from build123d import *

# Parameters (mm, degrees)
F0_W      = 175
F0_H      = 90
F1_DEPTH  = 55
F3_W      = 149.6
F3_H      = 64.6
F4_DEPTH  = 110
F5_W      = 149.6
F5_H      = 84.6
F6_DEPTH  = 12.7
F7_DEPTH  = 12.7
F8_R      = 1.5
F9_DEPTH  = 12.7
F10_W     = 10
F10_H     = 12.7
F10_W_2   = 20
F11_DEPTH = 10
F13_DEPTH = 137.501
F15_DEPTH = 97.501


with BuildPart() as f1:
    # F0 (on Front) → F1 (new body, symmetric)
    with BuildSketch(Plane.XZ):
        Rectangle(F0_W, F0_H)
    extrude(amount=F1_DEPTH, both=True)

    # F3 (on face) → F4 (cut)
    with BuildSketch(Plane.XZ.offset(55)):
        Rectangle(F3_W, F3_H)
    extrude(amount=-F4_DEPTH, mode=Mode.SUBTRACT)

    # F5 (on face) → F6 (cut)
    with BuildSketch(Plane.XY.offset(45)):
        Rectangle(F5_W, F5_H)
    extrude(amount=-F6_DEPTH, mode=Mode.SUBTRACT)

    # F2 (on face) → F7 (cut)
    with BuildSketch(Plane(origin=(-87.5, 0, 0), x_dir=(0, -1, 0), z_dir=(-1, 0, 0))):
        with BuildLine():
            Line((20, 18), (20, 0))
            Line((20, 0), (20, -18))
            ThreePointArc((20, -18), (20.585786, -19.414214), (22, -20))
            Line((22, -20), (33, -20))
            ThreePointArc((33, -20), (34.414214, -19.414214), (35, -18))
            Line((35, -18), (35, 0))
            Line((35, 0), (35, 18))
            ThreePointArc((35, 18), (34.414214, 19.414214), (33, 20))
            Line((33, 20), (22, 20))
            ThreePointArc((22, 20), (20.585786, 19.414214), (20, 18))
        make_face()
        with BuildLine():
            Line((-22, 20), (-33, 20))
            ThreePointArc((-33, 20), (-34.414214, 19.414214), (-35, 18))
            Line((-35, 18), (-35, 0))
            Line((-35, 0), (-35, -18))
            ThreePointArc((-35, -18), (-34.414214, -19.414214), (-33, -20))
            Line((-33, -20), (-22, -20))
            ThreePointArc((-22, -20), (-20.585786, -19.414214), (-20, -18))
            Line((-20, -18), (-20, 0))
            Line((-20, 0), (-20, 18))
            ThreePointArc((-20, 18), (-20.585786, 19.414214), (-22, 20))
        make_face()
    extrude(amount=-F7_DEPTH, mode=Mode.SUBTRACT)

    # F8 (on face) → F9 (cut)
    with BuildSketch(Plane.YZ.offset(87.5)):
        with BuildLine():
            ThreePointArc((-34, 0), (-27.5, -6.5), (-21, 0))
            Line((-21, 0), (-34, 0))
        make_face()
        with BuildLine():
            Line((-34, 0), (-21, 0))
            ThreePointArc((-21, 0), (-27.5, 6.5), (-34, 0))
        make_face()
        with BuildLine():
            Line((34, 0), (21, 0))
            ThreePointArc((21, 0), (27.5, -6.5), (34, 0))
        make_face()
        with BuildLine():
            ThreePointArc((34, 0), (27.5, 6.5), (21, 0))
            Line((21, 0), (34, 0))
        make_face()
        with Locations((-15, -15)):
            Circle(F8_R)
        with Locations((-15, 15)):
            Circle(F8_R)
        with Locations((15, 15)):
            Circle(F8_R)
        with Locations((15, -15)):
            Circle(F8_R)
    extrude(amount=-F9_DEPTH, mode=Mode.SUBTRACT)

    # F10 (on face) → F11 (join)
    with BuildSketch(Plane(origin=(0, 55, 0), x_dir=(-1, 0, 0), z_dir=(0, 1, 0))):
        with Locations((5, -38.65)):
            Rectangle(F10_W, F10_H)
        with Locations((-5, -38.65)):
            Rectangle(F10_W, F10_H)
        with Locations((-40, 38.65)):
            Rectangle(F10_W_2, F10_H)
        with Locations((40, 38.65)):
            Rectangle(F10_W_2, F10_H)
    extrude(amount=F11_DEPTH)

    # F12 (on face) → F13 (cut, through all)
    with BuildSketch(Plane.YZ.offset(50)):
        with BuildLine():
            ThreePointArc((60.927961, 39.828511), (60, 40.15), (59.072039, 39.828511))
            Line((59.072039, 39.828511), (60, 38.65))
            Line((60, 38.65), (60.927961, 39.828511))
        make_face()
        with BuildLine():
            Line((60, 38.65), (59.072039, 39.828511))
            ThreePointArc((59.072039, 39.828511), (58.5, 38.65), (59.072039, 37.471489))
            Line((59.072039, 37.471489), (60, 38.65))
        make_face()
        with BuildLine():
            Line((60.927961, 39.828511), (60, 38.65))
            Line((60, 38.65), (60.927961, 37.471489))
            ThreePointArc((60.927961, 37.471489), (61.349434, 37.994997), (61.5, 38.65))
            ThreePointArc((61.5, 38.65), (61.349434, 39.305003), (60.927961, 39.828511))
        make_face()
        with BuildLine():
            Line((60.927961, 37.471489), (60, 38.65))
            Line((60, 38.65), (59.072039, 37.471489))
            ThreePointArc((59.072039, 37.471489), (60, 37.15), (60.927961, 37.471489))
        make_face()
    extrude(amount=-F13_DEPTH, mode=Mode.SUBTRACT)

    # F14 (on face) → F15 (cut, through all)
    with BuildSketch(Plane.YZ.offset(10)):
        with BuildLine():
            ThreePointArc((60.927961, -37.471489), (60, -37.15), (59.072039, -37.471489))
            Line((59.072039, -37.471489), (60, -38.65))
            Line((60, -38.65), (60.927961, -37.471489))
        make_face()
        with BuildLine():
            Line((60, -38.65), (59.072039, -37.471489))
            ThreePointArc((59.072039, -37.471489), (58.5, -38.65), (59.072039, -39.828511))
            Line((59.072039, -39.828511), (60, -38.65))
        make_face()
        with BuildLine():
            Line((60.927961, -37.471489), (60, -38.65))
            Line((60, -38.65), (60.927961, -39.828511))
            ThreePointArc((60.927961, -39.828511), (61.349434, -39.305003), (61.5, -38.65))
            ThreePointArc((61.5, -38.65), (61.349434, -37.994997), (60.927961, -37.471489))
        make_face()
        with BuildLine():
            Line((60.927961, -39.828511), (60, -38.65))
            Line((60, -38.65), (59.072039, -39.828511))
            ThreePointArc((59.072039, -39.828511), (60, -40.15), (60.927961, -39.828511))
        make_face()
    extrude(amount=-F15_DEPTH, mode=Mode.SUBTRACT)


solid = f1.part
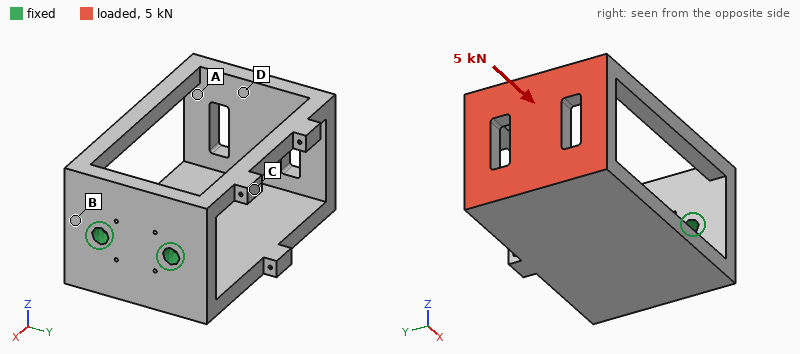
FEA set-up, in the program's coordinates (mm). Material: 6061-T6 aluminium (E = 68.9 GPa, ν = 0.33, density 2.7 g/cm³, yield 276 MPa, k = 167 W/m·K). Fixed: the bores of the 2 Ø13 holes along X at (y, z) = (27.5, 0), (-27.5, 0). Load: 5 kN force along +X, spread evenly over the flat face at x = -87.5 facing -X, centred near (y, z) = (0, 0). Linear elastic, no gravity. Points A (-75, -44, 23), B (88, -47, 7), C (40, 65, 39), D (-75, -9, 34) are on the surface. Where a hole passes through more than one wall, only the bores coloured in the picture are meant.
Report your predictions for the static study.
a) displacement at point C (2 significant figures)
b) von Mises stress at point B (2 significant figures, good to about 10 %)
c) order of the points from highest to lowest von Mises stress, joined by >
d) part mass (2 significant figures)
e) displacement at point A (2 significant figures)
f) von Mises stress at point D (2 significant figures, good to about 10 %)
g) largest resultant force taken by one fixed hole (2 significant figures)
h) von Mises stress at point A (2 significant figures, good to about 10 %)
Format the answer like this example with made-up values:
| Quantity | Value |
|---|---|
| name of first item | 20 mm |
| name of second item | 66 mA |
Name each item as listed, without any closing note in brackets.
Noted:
| Quantity | Value |
|---|---|
| displacement at point C | 0.072 mm |
| von Mises stress at point B | 21 MPa |
| order of the points from highest to lowest von Mises stress, joined by > | B > D > A > C |
| part mass | 1.3 kg |
| displacement at point A | 0.080 mm |
| von Mises stress at point D | 16 MPa |
| largest resultant force taken by one fixed hole | 2.5 kN |
| von Mises stress at point A | 12 MPa |
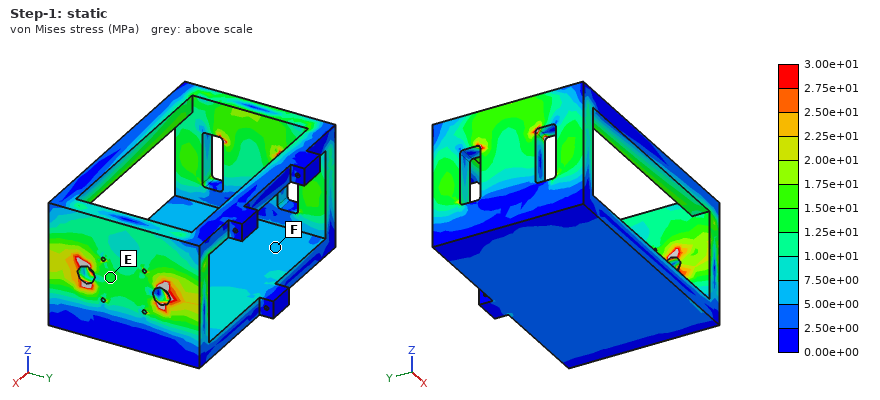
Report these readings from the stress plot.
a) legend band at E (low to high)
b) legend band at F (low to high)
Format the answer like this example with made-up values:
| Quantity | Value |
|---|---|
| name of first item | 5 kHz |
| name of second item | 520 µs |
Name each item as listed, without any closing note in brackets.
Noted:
| Quantity | Value |
|---|---|
| legend band at E | 1.25e+01 to 1.50e+01 MPa |
| legend band at F | 5.00e+00 to 7.50e+00 MPa |
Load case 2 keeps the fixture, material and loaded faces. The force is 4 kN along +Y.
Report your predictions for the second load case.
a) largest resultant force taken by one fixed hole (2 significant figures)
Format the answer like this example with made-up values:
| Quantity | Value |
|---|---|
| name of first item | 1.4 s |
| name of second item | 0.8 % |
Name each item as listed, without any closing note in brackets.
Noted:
| Quantity | Value |
|---|---|
| largest resultant force taken by one fixed hole | 9.3 kN |
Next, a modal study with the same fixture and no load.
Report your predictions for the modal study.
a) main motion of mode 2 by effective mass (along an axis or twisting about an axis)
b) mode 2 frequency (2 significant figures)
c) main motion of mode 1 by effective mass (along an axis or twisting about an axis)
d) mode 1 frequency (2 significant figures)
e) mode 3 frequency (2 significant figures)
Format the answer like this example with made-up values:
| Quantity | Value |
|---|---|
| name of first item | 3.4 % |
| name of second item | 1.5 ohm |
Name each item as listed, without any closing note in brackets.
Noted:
| Quantity | Value |
|---|---|
| main motion of mode 2 by effective mass | along Y |
| mode 2 frequency | 450 Hz |
| main motion of mode 1 by effective mass | along Z |
| mode 1 frequency | 290 Hz |
| mode 3 frequency | 850 Hz |
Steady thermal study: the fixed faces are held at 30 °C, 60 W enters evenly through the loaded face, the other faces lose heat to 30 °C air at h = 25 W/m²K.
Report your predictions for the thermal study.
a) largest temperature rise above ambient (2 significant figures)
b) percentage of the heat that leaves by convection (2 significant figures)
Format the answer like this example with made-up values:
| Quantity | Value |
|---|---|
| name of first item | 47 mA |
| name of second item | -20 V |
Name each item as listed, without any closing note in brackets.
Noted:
| Quantity | Value |
|---|---|
| largest temperature rise above ambient | 30 K |
| percentage of the heat that leaves by convection | 48 % |
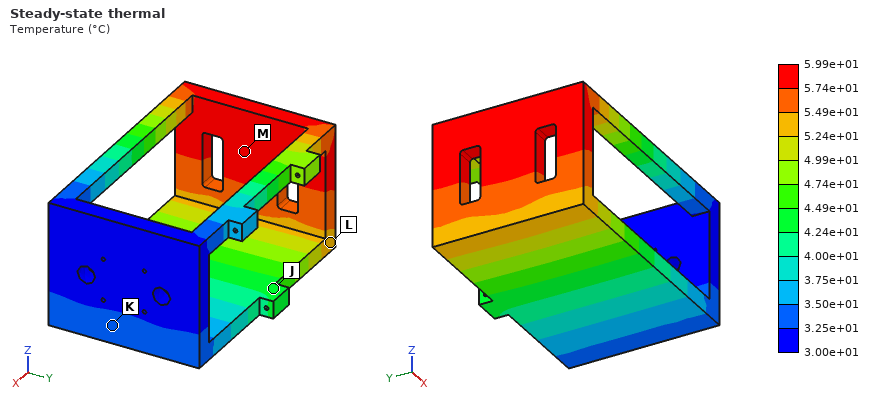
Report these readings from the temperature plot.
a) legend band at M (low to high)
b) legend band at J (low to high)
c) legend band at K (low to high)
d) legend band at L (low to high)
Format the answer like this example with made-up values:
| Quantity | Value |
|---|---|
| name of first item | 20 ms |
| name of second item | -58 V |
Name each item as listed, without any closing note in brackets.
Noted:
| Quantity | Value |
|---|---|
| legend band at M | 5.74e+01 to 5.99e+01 °C |
| legend band at J | 4.24e+01 to 4.49e+01 °C |
| legend band at K | 3.25e+01 to 3.50e+01 °C |
| legend band at L | 5.24e+01 to 5.49e+01 °C |
